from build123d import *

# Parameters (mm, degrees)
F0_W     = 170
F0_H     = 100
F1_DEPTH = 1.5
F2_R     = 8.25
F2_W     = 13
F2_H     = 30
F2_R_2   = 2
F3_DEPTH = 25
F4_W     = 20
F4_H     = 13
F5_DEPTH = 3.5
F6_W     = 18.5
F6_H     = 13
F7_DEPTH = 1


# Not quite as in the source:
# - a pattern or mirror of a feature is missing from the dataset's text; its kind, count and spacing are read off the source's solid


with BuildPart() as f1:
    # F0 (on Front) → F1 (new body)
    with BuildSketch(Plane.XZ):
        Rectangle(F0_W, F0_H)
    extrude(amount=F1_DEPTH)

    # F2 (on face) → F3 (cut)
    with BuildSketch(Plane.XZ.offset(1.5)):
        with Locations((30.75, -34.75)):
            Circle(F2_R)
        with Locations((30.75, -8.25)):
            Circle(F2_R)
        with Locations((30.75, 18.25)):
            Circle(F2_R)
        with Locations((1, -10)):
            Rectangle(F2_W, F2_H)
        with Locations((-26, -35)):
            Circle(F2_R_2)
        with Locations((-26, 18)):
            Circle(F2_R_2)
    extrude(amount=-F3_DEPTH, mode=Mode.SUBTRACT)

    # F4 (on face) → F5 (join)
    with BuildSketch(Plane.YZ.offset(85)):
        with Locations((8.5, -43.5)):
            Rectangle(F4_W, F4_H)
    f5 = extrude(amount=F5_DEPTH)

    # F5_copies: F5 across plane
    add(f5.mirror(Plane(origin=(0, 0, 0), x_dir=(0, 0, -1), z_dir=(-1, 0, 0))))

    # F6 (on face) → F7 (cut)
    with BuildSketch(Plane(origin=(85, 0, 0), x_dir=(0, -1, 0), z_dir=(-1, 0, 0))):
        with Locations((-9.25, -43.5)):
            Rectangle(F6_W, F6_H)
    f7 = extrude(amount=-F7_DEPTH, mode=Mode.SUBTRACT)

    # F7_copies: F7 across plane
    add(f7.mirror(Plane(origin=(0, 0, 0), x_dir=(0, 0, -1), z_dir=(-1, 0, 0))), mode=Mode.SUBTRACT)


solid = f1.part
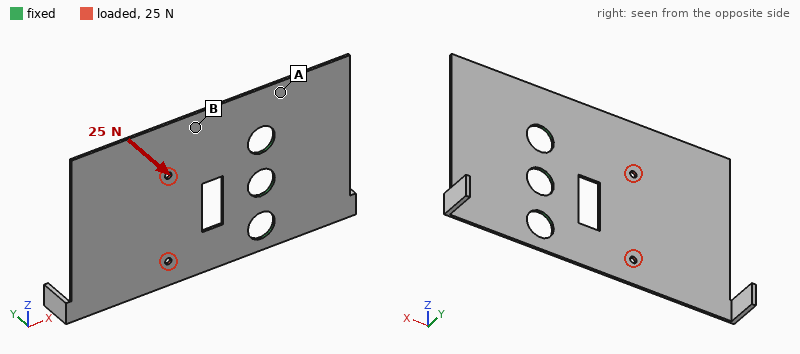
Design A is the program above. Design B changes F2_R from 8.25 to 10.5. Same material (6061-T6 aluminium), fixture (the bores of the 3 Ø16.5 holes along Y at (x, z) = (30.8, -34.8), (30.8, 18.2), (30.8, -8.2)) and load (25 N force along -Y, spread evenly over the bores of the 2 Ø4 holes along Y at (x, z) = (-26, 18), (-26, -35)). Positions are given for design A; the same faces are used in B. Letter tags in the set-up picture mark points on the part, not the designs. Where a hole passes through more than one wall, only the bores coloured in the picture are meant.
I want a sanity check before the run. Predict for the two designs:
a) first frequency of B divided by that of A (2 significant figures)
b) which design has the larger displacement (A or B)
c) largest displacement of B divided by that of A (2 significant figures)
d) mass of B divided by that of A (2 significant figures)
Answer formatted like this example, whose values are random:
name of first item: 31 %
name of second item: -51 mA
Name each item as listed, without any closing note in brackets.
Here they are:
first frequency of B divided by that of A: 1.0
which design has the larger displacement: A
largest displacement of B divided by that of A: 0.91
mass of B divided by that of A: 0.98
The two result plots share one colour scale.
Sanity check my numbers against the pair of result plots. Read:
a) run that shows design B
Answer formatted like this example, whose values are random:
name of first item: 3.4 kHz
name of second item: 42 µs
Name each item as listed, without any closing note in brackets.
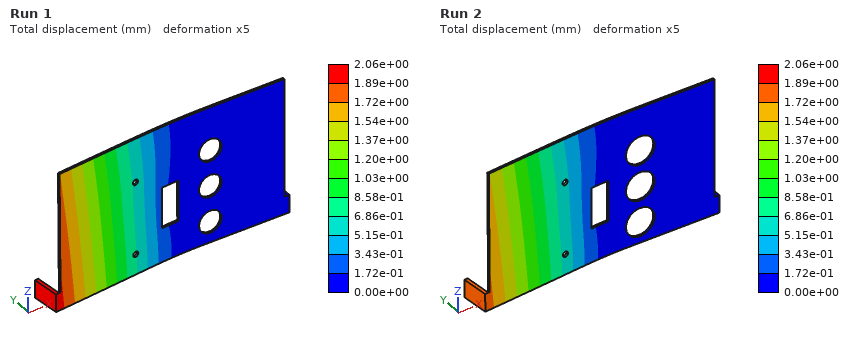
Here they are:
run that shows design B: Run 2
